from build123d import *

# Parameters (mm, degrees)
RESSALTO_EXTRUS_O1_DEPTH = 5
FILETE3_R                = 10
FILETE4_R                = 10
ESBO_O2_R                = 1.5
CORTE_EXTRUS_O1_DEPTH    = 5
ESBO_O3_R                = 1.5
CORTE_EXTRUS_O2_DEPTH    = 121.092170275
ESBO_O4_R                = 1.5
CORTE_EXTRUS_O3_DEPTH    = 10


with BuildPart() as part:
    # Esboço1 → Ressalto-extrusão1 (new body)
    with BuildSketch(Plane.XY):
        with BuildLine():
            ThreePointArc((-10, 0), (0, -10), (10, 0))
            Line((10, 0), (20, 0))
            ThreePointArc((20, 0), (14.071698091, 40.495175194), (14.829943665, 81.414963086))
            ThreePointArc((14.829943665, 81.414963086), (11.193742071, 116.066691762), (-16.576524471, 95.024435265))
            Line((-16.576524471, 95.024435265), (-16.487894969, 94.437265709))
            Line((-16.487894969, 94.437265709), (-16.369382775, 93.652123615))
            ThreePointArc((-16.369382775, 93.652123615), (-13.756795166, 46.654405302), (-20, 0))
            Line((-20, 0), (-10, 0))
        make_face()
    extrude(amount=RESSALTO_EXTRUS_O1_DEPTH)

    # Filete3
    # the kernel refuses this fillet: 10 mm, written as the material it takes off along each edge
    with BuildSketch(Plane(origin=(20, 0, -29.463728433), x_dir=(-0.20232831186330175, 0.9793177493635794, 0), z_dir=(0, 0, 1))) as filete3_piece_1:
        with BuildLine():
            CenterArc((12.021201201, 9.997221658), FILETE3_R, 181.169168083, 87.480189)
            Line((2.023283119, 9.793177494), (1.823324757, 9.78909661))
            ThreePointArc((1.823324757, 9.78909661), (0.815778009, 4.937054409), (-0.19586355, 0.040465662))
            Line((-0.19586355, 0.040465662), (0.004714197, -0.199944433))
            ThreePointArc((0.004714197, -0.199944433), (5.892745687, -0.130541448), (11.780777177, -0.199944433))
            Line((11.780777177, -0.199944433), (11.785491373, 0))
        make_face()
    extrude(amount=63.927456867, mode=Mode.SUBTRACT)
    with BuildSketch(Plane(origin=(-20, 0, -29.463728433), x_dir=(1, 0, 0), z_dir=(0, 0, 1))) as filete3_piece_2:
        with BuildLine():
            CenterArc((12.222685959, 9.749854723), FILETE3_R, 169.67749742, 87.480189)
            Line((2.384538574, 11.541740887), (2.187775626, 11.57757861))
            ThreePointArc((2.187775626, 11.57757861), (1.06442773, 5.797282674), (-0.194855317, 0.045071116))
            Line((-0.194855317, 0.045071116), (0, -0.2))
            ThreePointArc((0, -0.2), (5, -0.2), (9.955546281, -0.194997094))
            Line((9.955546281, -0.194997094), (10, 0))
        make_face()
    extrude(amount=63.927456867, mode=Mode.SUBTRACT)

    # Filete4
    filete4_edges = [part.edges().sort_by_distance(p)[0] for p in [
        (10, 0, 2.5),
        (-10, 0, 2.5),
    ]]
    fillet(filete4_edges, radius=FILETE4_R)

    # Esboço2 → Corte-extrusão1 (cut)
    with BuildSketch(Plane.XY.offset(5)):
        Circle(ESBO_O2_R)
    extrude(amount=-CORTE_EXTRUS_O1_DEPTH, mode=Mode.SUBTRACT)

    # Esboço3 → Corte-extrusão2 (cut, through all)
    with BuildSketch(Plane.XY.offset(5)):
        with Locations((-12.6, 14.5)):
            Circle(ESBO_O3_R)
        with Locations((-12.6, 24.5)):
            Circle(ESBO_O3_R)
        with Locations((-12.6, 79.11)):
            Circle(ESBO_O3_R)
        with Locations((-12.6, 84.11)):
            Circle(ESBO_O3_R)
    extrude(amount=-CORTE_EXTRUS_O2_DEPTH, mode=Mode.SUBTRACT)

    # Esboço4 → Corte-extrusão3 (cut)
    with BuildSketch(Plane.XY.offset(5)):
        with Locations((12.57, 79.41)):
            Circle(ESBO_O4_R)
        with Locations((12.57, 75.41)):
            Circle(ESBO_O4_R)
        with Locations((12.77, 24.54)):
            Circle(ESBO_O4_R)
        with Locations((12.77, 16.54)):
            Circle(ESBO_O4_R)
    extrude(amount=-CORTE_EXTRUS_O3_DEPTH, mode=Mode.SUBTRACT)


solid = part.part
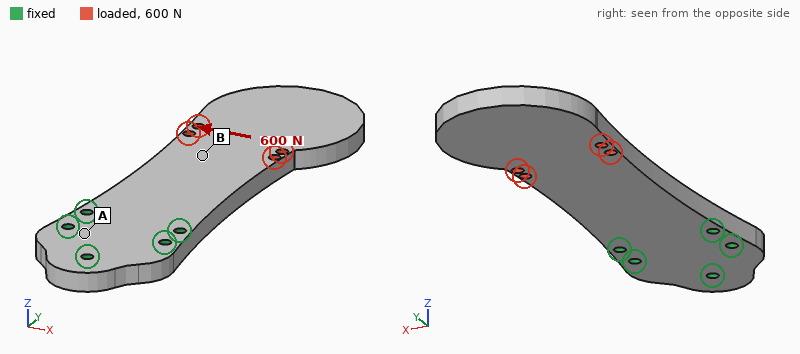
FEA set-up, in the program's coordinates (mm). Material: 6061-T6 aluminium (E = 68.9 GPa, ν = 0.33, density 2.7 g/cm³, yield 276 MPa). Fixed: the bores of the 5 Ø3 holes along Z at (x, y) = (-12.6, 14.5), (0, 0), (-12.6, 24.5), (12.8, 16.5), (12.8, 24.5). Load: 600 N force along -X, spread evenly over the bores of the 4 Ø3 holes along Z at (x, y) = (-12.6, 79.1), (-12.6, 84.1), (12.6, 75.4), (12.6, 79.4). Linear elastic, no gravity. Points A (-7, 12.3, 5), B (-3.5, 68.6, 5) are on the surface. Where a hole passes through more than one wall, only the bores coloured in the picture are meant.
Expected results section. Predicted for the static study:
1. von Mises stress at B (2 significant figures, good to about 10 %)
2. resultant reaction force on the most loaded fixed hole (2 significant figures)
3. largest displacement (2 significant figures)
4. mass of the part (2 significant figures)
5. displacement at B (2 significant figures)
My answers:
11 MPa
1.2 kN
0.11 mm
50 g
0.041 mm
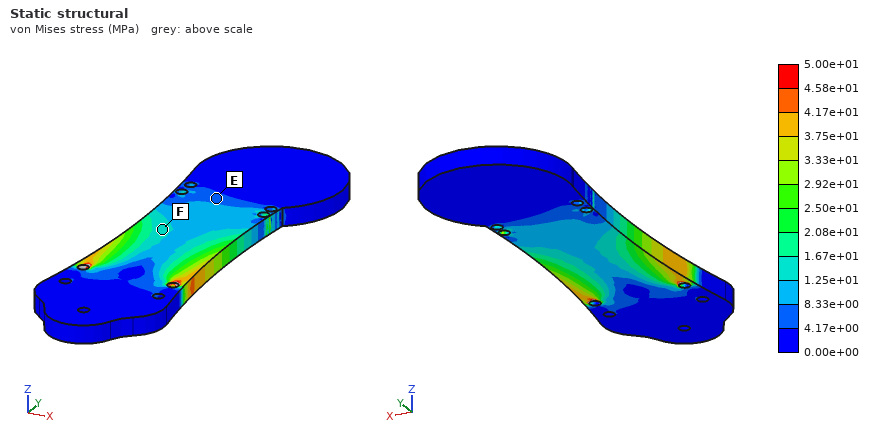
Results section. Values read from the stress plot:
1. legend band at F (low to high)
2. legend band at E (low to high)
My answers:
1.25e+01 to 1.67e+01 MPa
4.17e+00 to 8.33e+00 MPa
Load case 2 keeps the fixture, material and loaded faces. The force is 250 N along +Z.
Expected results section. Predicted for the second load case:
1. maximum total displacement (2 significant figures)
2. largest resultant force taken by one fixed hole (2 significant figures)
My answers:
1.4 mm
380 N
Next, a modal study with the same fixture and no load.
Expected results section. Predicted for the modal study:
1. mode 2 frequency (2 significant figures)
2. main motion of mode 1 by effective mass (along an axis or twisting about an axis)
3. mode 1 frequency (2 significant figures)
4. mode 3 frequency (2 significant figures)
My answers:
2300 Hz
along Z
440 Hz
2400 Hz
